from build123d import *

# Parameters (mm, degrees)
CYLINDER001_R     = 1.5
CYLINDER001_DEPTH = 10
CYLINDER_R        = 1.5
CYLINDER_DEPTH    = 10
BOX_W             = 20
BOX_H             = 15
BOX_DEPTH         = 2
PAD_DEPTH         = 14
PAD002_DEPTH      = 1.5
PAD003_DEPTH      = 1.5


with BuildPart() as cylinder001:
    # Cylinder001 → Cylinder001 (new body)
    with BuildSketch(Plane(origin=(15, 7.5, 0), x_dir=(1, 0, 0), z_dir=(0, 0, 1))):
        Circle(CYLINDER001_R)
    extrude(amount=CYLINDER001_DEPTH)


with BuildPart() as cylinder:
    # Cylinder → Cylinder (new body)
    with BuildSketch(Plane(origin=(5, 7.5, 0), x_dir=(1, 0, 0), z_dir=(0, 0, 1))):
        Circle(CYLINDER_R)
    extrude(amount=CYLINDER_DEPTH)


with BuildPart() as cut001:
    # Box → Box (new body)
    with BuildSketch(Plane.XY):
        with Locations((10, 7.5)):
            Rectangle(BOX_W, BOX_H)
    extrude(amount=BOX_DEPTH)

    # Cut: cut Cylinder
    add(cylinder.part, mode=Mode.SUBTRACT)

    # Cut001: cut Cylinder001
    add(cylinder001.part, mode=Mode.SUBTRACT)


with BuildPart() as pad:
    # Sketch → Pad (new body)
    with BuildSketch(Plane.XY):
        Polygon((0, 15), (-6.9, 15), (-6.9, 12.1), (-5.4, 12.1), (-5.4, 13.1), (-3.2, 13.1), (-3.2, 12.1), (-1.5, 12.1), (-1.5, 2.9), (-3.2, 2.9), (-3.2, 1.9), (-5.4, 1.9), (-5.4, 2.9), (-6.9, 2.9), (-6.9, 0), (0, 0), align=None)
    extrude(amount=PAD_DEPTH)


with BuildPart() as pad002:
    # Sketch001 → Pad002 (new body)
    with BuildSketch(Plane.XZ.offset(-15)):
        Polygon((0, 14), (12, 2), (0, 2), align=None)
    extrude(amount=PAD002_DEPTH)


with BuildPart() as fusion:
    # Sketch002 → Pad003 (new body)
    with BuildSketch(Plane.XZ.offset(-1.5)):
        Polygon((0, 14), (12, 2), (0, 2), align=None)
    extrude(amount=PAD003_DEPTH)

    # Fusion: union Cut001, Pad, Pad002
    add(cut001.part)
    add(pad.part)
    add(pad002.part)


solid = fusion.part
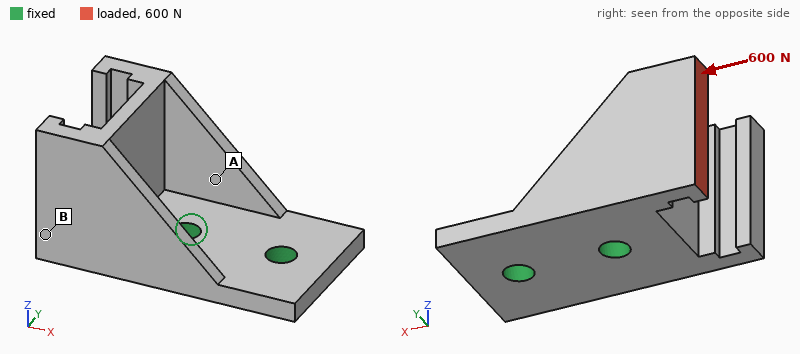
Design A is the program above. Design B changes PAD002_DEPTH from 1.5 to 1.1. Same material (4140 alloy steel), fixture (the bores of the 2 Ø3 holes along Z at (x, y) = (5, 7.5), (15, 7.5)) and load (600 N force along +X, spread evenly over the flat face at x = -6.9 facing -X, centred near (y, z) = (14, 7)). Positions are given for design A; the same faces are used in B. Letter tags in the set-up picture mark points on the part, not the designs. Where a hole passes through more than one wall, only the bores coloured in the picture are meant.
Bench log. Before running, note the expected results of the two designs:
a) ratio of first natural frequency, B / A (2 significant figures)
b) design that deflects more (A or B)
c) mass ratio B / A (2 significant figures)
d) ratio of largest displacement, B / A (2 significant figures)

0.99
B
0.98
1.1
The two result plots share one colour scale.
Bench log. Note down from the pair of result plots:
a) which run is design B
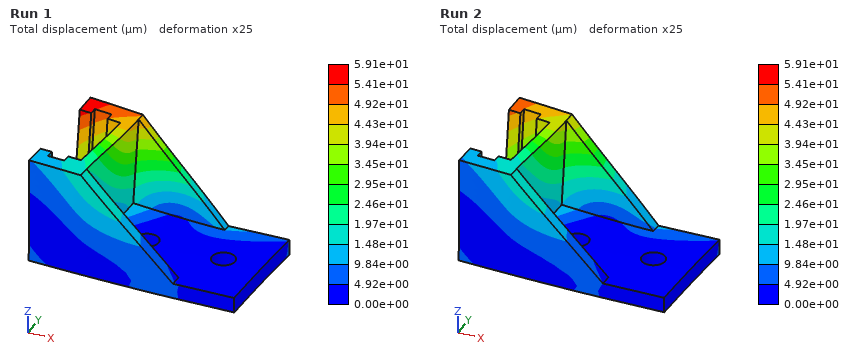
Run 1
